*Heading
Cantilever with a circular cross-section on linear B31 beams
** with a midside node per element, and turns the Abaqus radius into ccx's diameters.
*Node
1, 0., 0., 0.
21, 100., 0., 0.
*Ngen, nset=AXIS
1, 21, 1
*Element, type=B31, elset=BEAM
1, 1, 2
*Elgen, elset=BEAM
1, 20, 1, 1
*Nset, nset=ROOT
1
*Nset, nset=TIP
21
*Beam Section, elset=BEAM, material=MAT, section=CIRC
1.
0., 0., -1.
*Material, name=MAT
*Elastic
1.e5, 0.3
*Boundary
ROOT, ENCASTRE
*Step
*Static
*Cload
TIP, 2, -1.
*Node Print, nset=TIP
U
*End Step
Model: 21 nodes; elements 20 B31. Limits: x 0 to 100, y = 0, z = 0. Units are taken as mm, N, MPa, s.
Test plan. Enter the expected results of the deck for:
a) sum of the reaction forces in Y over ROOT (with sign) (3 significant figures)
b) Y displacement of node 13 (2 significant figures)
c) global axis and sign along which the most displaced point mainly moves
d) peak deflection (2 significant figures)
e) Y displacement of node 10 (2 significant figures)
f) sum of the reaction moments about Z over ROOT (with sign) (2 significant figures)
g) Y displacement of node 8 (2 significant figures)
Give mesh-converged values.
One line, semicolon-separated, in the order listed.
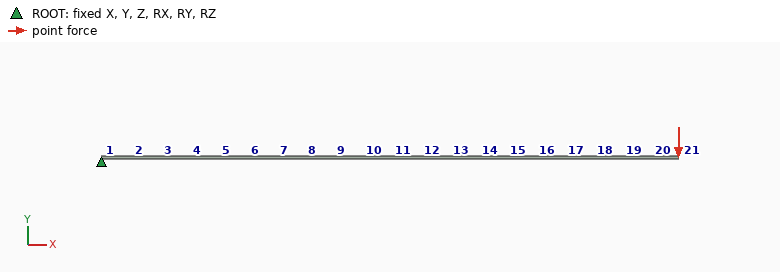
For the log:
1.00 N; -1.8 mm; -Y; 4.2 mm; -1.1 mm; 100 N·mm; -0.69 mm
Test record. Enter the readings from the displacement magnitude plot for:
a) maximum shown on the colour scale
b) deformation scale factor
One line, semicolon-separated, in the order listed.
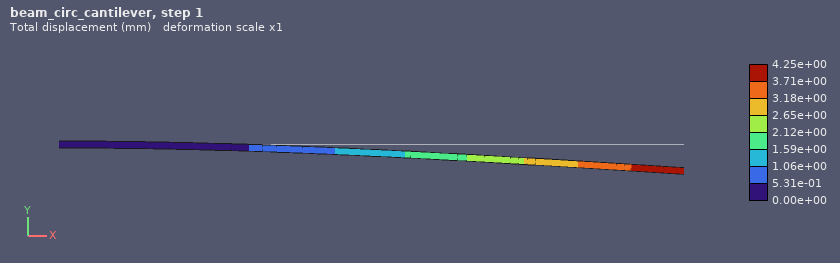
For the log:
4.25e+00 mm; 1
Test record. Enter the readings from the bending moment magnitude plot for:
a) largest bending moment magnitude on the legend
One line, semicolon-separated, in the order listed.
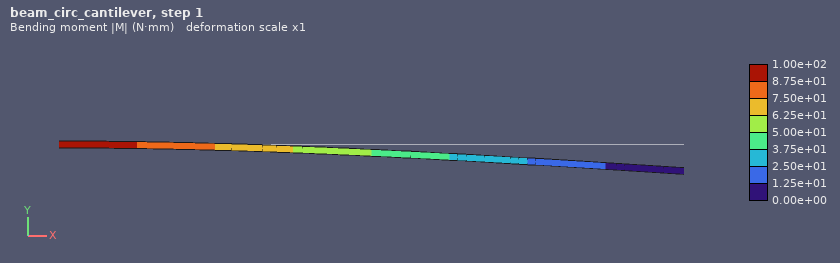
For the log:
1.00e+02 N·mm
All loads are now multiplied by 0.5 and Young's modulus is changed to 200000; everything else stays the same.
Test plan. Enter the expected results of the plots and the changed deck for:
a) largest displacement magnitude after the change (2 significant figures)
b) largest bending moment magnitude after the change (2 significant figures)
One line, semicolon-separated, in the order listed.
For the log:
1.1 mm; 50 N·mm
